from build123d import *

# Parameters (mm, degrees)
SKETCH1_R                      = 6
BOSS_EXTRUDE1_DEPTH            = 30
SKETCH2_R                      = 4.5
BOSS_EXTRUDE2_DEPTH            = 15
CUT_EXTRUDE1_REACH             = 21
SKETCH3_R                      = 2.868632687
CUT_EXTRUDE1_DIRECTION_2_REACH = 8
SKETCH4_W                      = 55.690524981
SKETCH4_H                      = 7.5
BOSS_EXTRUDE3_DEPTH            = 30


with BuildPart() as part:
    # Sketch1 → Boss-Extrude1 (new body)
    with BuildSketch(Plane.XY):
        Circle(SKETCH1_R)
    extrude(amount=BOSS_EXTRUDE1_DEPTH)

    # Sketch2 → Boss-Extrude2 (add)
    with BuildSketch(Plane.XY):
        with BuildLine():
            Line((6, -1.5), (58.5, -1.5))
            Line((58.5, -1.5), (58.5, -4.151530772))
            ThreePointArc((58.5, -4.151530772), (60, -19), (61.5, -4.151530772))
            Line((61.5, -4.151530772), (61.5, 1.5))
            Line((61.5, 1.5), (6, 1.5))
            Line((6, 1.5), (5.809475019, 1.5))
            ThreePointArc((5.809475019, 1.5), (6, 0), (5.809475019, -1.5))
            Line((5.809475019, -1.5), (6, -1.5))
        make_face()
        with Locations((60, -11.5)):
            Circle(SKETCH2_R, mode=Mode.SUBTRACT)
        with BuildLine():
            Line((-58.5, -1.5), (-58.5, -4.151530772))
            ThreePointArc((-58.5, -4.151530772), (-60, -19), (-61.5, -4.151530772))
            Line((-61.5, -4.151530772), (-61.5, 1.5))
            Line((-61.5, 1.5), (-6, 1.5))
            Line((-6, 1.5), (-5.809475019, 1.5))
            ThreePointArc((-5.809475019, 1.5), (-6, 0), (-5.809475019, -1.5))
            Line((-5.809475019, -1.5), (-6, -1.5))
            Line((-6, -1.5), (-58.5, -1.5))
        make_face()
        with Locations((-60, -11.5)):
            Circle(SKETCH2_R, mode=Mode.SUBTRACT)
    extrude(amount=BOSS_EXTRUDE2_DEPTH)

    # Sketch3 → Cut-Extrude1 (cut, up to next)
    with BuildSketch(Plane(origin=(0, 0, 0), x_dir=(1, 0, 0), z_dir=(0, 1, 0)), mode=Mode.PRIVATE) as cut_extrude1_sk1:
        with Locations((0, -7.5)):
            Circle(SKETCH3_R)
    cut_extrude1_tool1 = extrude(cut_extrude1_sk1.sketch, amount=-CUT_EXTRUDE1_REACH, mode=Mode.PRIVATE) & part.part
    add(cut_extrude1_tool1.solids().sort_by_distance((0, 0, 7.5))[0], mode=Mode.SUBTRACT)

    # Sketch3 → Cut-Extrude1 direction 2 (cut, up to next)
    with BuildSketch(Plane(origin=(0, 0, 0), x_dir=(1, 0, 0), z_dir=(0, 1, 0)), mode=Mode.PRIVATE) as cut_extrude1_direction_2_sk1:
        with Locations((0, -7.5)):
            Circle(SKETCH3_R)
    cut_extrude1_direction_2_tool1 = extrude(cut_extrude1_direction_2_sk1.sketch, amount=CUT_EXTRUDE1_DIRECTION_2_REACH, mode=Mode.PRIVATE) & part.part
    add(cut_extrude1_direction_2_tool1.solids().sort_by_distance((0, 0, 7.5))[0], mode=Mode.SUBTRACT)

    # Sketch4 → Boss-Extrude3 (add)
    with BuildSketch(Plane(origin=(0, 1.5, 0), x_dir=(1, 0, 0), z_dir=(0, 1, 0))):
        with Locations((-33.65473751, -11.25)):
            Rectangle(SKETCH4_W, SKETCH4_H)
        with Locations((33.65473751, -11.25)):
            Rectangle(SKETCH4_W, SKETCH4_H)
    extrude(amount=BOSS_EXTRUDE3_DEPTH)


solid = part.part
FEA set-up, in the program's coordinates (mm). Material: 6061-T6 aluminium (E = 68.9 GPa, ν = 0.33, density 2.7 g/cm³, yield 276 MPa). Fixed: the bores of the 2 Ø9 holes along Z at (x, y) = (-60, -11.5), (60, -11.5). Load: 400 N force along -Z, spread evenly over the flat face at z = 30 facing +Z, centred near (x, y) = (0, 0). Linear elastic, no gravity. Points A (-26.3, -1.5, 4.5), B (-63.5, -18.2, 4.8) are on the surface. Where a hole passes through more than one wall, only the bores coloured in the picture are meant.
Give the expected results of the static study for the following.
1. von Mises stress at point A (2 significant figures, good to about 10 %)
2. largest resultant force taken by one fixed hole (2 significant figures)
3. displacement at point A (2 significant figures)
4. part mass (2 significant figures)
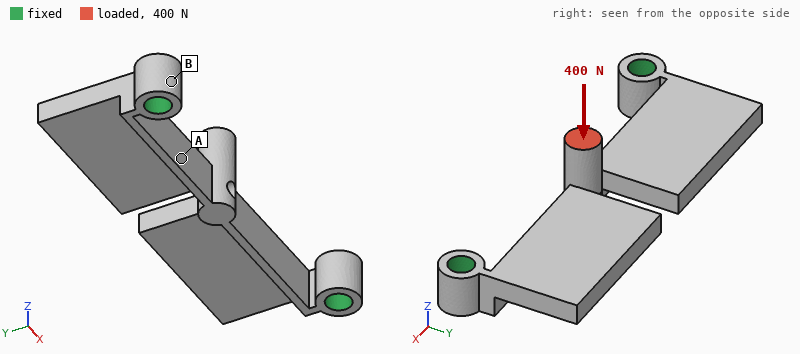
12 MPa
200 N
66 µm
99 g
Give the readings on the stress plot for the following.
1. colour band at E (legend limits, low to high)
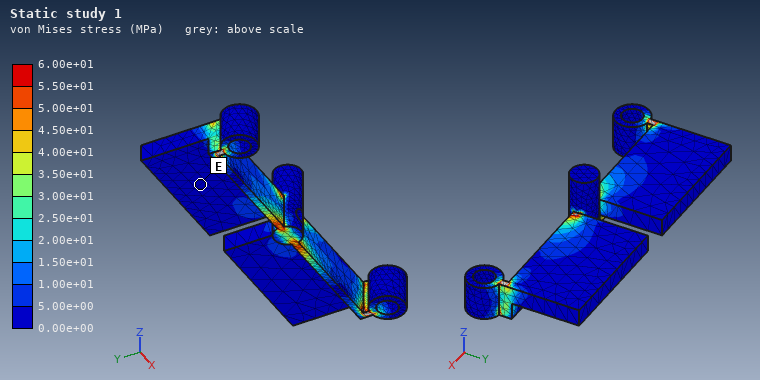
0.00e+00 to 5.00e+00 MPa
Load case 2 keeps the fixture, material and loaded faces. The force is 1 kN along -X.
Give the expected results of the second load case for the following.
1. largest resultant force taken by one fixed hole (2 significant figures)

540 N
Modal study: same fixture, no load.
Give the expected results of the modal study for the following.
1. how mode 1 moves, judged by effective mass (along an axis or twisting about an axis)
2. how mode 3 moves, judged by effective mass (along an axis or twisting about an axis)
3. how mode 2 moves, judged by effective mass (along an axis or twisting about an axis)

along Y
twisting about Y
along Z
